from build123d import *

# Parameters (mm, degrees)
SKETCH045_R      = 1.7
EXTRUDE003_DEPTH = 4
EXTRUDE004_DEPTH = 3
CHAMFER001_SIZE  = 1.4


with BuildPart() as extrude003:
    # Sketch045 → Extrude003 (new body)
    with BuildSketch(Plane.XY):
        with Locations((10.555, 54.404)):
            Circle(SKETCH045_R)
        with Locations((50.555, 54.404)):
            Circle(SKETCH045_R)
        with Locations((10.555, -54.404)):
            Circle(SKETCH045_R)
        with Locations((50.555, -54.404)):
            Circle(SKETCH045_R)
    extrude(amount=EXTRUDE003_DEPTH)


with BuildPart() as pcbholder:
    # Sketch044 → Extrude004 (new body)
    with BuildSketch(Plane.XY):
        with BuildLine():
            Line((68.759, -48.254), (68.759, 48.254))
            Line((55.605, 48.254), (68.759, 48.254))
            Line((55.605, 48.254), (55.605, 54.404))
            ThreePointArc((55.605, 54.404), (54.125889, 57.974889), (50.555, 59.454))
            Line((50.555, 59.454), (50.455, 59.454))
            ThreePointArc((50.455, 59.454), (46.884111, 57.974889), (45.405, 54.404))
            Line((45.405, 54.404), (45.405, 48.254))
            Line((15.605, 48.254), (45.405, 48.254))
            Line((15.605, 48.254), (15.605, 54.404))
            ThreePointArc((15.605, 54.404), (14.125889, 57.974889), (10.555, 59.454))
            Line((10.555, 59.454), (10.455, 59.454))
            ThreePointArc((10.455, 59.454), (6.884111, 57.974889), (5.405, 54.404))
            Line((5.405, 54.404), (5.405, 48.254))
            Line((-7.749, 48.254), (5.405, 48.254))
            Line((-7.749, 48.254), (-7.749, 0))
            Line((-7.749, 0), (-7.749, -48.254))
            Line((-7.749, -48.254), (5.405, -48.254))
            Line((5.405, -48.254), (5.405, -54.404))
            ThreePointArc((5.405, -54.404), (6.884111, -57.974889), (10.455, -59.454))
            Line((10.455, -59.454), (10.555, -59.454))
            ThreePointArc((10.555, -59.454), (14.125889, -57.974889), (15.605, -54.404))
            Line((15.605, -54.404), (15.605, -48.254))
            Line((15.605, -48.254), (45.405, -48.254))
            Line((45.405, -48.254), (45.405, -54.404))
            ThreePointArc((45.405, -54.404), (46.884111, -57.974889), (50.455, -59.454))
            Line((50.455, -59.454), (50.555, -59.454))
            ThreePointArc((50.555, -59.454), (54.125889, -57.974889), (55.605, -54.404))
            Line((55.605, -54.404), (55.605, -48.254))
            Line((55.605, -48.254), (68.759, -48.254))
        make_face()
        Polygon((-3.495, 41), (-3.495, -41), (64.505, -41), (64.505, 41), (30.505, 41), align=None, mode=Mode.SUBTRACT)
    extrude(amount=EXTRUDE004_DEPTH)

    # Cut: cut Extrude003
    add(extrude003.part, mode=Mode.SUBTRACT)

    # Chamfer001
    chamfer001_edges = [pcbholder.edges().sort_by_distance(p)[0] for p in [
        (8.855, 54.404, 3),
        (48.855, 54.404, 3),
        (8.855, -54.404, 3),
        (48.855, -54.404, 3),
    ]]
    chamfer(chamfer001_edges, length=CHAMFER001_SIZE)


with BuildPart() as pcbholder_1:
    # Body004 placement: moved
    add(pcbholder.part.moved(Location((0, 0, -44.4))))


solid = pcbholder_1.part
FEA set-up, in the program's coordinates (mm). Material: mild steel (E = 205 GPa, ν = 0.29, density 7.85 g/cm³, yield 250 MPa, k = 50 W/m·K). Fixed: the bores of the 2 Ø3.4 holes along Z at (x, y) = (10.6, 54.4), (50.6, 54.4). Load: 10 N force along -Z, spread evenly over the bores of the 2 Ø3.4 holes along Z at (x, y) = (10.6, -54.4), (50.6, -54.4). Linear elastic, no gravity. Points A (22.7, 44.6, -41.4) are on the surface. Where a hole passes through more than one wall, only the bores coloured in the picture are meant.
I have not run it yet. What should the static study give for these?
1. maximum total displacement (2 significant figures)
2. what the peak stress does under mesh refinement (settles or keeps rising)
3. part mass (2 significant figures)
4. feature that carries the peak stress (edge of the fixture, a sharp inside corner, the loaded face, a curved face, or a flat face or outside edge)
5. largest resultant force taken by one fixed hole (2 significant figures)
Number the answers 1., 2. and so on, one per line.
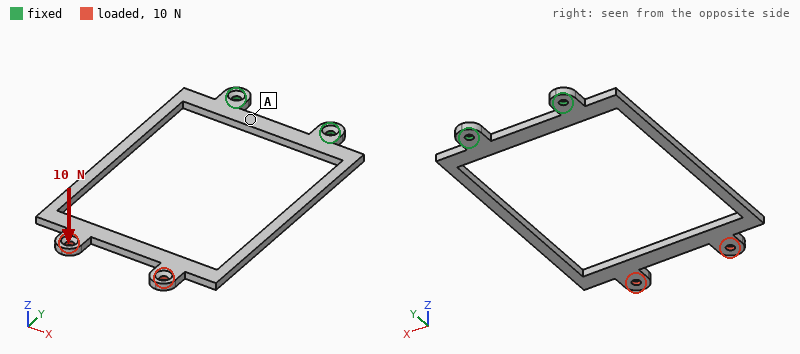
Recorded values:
1. 1.2 mm
2. keeps rising
3. 51 g
4. edge of the fixture
5. 5.0 N
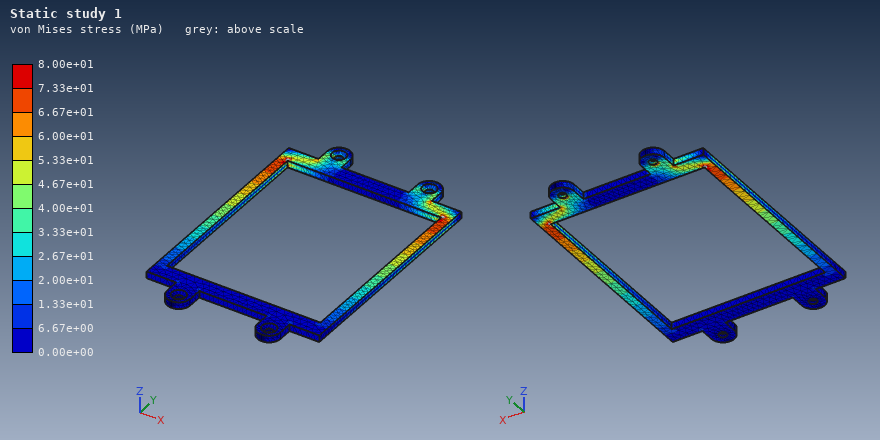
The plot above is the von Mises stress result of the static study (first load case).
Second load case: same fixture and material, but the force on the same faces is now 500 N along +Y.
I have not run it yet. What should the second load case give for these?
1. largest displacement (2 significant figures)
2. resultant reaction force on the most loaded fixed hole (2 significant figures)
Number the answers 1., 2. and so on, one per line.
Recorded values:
1. 0.57 mm
2. 420 N
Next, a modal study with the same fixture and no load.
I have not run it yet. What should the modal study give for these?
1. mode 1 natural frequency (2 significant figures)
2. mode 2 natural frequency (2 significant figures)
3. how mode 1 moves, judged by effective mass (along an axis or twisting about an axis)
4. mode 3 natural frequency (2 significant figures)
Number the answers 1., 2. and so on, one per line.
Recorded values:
1. 120 Hz
2. 350 Hz
3. along Z
4. 350 Hz
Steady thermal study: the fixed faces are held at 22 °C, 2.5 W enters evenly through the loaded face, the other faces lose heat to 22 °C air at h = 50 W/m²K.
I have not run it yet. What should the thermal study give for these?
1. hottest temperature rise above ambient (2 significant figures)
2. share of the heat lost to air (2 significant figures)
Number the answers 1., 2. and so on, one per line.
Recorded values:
1. 26 K
2. 98 %
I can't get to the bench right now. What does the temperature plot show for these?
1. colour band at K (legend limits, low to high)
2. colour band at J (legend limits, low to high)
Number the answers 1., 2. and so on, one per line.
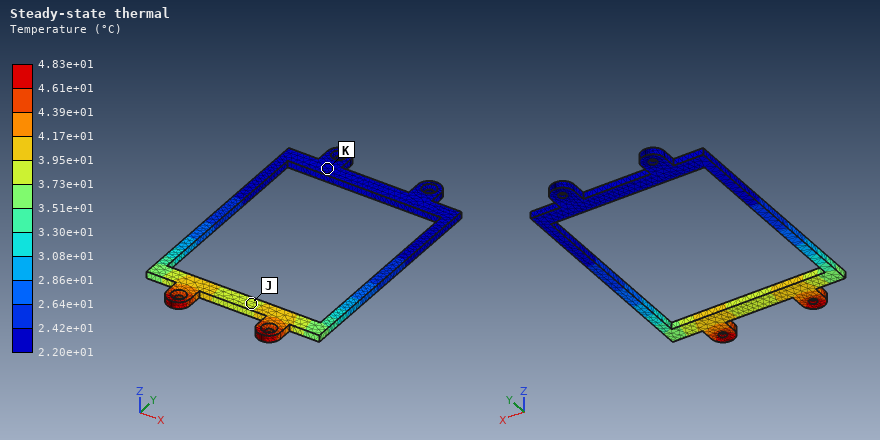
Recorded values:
1. 2.20e+01 to 2.42e+01 °C
2. 3.73e+01 to 3.95e+01 °C
